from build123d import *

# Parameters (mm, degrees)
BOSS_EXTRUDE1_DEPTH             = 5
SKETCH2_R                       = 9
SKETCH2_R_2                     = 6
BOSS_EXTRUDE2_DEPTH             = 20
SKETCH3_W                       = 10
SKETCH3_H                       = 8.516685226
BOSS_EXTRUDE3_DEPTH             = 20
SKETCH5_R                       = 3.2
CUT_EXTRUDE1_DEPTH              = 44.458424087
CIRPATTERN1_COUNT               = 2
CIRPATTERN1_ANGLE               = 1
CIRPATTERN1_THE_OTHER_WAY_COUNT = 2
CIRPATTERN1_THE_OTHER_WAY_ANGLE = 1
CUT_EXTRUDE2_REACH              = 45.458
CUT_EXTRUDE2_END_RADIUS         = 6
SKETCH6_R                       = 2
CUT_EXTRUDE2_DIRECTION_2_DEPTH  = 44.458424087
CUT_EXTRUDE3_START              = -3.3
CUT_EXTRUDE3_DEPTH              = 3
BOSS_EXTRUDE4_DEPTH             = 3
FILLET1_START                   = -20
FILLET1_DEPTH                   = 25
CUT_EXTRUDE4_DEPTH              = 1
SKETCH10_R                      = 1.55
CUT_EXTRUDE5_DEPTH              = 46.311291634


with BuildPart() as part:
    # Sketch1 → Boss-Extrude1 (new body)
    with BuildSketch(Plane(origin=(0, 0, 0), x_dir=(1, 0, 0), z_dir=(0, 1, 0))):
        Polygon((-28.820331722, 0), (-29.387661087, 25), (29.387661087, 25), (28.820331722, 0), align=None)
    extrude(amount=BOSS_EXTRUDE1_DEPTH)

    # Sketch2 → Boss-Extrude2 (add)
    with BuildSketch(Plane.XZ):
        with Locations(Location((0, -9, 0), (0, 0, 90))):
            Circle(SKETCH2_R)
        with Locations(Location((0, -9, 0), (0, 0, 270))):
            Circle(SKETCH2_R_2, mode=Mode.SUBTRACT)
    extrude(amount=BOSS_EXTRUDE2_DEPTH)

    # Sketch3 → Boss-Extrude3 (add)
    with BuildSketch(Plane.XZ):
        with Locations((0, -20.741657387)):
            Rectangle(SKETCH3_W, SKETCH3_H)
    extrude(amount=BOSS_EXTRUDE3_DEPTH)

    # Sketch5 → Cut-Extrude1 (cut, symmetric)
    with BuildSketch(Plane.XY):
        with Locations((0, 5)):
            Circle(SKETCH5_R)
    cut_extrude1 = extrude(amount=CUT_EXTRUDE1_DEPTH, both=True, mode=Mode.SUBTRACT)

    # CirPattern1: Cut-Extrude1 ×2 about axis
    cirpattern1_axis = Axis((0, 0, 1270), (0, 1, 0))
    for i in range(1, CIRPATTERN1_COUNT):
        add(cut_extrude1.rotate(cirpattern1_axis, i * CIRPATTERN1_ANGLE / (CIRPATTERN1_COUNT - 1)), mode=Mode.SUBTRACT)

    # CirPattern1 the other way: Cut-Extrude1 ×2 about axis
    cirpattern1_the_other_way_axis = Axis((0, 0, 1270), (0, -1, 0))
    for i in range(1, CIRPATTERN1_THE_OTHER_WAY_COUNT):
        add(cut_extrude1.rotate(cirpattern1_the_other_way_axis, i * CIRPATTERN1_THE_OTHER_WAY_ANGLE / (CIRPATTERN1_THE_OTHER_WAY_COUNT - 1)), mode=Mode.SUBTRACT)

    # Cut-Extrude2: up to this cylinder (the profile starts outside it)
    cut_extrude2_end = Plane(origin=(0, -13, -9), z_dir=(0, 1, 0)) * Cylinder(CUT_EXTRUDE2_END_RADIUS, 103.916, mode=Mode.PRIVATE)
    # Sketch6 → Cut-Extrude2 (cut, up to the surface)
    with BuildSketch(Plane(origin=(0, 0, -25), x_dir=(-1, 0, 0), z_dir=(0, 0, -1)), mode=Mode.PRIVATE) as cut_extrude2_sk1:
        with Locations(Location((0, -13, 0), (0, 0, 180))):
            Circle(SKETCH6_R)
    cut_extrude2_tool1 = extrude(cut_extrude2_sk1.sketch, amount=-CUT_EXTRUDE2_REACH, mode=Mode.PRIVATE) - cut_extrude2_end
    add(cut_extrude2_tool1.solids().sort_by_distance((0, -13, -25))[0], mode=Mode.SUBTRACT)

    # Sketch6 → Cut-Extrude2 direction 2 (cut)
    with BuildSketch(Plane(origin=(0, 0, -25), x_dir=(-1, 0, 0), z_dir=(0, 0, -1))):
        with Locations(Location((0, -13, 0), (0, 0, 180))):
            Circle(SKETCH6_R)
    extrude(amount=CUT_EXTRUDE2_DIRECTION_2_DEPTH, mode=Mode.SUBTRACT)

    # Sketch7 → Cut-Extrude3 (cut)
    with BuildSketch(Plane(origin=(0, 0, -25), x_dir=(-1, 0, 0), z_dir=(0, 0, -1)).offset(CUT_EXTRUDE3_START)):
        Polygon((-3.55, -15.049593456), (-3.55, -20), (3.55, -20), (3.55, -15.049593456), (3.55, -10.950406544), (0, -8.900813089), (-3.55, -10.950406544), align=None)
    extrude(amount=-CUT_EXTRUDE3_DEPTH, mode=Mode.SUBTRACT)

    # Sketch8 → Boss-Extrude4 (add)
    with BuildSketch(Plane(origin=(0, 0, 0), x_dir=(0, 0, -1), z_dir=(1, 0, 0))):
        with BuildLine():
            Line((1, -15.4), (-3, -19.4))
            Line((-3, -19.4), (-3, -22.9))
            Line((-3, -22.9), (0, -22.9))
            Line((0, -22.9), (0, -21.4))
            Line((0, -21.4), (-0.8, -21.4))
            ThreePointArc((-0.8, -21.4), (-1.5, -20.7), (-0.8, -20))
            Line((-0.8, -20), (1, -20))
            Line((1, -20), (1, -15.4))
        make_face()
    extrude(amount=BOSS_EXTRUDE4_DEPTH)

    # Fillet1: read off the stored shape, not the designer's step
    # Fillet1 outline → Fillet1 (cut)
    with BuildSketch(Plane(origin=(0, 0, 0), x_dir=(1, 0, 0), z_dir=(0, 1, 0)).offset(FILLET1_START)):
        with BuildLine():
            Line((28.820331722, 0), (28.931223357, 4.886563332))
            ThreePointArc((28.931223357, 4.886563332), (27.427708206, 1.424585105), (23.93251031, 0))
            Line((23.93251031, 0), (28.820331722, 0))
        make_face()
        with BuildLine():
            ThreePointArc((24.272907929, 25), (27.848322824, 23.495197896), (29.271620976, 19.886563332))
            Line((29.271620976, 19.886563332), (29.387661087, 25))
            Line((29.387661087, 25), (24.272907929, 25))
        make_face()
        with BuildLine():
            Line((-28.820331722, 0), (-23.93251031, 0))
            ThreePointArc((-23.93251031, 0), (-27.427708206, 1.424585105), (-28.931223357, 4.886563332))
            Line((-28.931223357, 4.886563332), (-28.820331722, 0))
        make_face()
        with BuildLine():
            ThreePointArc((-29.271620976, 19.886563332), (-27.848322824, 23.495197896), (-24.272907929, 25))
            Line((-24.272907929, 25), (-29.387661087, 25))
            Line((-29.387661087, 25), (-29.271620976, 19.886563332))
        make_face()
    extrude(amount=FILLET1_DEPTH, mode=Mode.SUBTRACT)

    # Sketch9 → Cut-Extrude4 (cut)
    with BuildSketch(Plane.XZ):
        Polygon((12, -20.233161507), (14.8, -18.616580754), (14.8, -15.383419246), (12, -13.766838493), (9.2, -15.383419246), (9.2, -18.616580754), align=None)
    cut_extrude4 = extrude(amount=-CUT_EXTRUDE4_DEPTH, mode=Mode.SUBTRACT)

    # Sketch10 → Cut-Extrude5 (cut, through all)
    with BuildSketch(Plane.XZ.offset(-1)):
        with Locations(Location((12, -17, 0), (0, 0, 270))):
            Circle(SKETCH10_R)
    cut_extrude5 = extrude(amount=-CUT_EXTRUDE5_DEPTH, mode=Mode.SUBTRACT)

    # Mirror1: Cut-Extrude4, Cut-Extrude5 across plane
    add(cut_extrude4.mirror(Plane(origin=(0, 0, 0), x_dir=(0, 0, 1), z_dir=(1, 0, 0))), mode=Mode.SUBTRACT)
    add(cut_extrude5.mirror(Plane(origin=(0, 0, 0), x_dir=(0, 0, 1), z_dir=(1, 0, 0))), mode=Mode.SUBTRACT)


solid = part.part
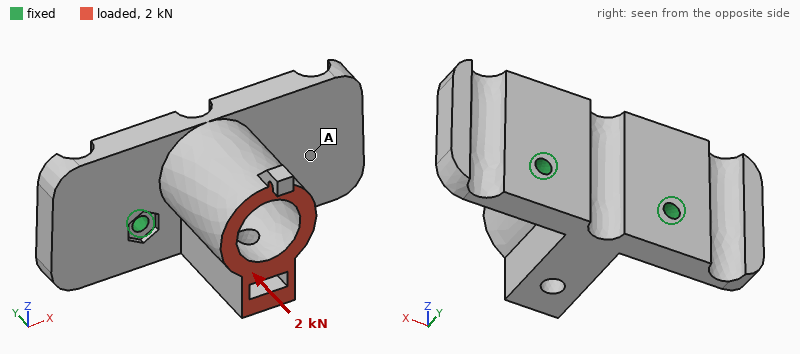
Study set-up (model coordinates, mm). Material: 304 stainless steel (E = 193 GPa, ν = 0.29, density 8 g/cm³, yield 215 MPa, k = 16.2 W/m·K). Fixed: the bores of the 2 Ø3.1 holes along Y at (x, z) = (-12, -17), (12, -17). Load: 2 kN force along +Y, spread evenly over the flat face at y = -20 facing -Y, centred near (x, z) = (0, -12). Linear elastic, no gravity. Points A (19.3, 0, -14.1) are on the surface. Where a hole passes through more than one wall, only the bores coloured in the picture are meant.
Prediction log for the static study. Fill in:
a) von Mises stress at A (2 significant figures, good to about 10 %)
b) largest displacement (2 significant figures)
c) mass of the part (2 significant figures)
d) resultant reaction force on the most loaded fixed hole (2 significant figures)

17 MPa
28 µm
79 g
1.1 kN
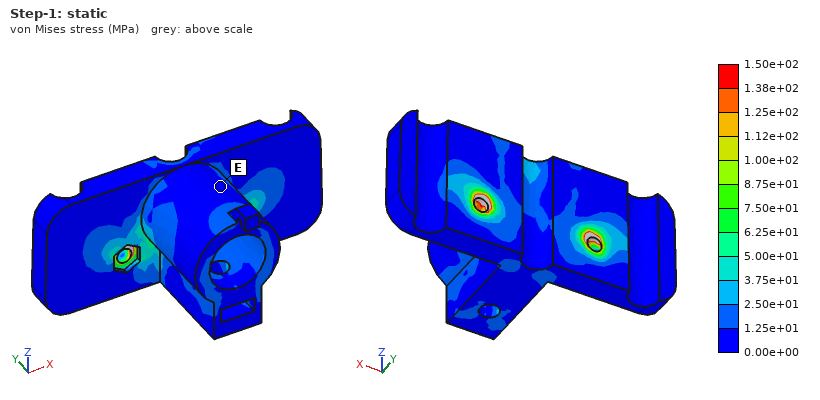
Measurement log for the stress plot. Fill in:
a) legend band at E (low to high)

0.00e+00 to 1.25e+01 MPa
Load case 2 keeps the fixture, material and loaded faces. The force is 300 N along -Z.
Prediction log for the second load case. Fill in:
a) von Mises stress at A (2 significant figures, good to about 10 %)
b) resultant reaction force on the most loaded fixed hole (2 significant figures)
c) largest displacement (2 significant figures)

11 MPa
210 N
23 µm
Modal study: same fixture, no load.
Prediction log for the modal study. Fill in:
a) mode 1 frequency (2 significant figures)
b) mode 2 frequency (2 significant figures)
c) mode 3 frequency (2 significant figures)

4900 Hz
8400 Hz
8500 Hz
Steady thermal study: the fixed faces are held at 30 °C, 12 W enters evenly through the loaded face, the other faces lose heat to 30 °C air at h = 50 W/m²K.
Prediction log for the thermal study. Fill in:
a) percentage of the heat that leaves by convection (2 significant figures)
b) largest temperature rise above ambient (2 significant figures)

59 %
74 K
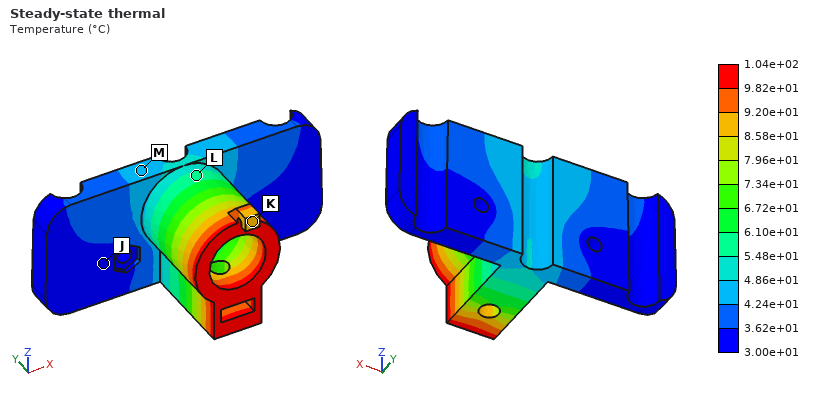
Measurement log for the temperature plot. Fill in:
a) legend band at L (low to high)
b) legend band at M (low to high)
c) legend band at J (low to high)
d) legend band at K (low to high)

5.48e+01 to 6.10e+01 °C
4.24e+01 to 4.86e+01 °C
3.00e+01 to 3.62e+01 °C
8.58e+01 to 9.20e+01 °C
